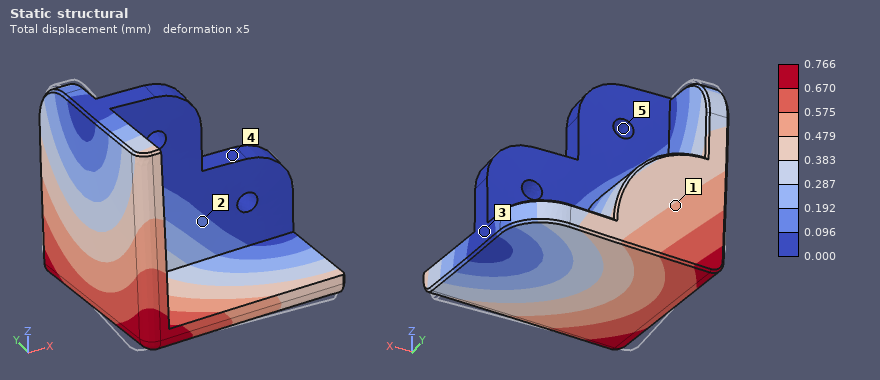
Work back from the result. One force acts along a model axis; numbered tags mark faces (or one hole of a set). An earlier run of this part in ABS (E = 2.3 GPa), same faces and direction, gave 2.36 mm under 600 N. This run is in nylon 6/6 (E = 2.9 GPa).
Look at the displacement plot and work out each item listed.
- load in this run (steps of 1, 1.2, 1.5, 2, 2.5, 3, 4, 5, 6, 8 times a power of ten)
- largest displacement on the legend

250 N
0.766 mm
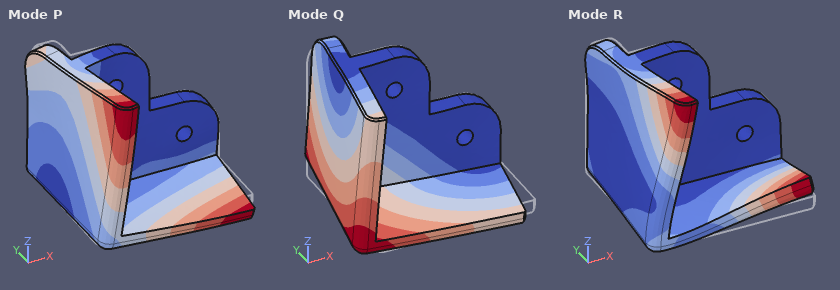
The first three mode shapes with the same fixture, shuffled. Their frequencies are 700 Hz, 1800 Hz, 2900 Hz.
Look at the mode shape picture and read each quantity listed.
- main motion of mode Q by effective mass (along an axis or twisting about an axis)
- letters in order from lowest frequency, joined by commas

along Y
Q, P, R
